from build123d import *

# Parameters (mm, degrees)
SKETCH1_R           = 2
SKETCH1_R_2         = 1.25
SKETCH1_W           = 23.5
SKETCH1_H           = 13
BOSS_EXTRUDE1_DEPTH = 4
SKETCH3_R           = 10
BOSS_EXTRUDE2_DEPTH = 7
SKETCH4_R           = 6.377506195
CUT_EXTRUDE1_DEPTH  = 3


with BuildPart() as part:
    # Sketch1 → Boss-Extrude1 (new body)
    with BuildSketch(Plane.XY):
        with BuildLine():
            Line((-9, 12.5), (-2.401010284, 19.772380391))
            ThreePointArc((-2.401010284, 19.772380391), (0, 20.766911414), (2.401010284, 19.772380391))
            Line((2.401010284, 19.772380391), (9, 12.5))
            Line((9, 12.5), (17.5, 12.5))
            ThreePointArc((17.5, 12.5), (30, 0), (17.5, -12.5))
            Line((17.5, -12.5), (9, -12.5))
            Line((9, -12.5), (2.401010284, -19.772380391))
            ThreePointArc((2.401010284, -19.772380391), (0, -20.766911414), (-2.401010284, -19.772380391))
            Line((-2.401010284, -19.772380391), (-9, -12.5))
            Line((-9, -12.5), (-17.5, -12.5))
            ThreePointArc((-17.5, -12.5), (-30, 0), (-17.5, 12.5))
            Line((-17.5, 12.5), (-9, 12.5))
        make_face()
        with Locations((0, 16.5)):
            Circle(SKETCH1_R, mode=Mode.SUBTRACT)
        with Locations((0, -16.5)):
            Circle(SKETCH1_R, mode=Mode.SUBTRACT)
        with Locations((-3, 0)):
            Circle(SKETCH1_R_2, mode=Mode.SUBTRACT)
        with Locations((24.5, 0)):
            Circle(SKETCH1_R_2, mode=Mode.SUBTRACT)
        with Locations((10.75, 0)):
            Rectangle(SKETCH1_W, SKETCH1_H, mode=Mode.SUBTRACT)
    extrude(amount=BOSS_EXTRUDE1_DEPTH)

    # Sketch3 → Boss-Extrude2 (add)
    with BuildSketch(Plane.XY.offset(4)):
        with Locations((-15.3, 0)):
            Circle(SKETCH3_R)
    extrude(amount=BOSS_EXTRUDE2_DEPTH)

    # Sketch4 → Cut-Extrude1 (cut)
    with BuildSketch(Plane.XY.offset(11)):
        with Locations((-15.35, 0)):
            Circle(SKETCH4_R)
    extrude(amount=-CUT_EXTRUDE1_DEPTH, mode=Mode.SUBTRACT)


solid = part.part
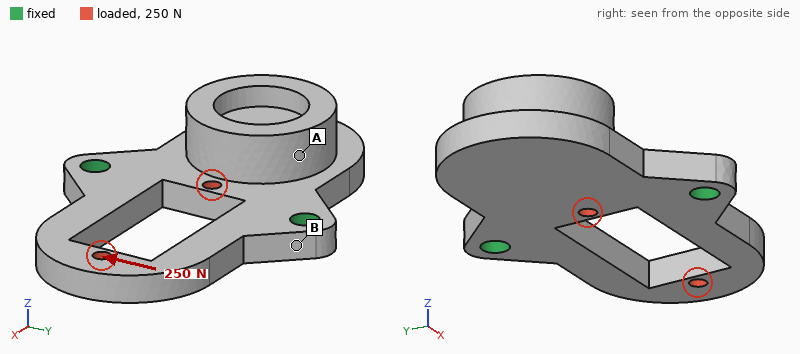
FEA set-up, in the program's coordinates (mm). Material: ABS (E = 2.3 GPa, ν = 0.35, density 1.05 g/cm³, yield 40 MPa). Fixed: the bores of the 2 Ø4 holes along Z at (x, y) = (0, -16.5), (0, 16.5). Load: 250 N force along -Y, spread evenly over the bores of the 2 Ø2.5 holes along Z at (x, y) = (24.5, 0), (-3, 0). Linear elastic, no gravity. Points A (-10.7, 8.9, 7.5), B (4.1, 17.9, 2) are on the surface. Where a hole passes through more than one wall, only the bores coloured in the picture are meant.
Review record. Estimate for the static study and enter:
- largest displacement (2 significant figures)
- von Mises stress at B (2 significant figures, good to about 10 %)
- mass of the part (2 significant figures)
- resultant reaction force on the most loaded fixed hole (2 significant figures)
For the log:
0.46 mm
6.0 MPa
6.9 g
140 N
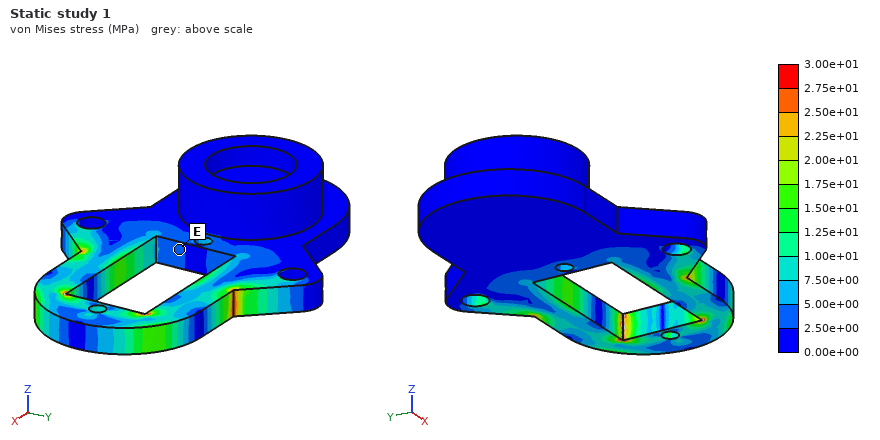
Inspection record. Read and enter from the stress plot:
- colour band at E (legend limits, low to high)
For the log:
2.50e+00 to 5.00e+00 MPa
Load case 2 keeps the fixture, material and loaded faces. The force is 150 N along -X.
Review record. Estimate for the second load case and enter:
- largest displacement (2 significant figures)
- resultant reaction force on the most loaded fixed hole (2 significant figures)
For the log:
59 µm
78 N
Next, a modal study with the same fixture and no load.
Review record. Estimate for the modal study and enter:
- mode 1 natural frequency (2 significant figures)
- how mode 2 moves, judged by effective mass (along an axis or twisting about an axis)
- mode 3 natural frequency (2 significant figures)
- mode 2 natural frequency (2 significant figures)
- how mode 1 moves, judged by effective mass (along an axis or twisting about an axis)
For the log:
850 Hz
along Z
2900 Hz
1100 Hz
along Z
